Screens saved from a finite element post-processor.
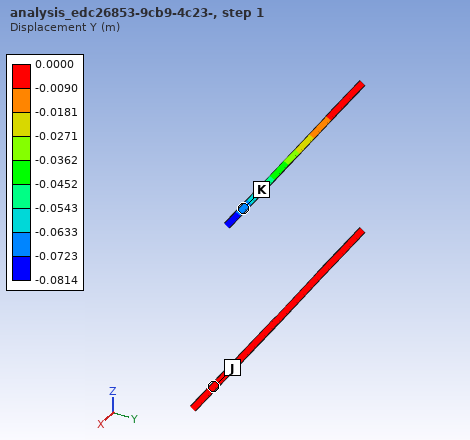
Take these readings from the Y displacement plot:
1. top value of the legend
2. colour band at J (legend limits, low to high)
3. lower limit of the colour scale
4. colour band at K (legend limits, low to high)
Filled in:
0.0000 m
-0.0090 to 0.0000 m
-0.0814 m
-0.0723 to -0.0633 m
